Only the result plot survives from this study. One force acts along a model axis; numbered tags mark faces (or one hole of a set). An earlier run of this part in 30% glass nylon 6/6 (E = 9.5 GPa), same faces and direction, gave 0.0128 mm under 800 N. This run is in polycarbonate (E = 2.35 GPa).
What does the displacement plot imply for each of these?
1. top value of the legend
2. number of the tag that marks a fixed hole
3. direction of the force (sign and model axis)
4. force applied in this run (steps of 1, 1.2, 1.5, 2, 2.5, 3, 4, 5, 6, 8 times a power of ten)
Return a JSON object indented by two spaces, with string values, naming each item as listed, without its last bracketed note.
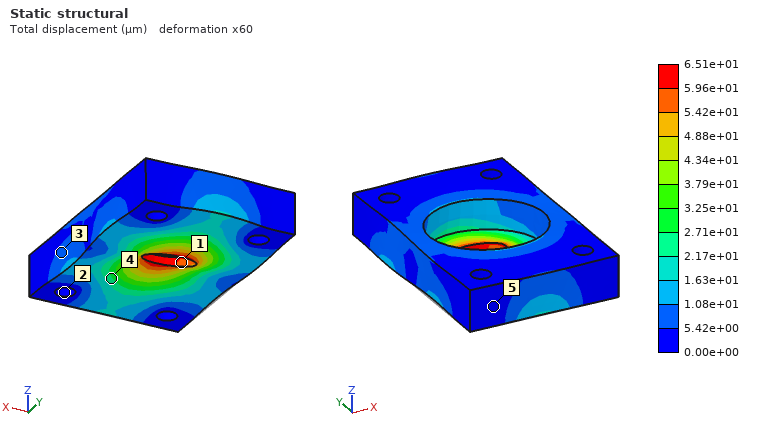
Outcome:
{
  "top value of the legend": "6.51e+01 µm",
  "number of the tag that marks a fixed hole": "2",
  "direction of the force": "+Y",
  "force applied in this run": "1 kN"
}
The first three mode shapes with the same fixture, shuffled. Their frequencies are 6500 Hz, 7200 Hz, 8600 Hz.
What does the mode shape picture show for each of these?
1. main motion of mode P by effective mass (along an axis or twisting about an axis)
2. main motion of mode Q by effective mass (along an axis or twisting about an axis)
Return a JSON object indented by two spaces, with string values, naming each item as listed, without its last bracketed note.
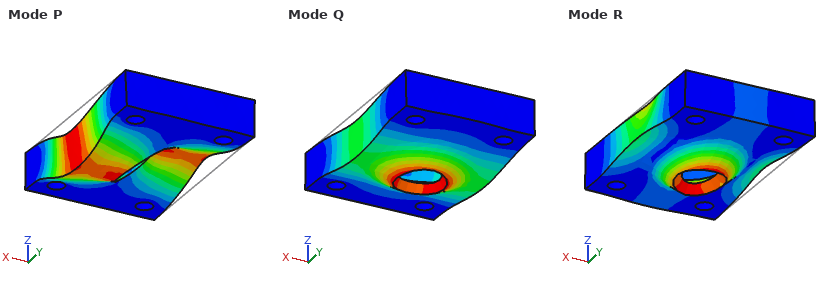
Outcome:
{
  "main motion of mode P by effective mass": "twisting about Y",
  "main motion of mode Q by effective mass": "along Z"
}
